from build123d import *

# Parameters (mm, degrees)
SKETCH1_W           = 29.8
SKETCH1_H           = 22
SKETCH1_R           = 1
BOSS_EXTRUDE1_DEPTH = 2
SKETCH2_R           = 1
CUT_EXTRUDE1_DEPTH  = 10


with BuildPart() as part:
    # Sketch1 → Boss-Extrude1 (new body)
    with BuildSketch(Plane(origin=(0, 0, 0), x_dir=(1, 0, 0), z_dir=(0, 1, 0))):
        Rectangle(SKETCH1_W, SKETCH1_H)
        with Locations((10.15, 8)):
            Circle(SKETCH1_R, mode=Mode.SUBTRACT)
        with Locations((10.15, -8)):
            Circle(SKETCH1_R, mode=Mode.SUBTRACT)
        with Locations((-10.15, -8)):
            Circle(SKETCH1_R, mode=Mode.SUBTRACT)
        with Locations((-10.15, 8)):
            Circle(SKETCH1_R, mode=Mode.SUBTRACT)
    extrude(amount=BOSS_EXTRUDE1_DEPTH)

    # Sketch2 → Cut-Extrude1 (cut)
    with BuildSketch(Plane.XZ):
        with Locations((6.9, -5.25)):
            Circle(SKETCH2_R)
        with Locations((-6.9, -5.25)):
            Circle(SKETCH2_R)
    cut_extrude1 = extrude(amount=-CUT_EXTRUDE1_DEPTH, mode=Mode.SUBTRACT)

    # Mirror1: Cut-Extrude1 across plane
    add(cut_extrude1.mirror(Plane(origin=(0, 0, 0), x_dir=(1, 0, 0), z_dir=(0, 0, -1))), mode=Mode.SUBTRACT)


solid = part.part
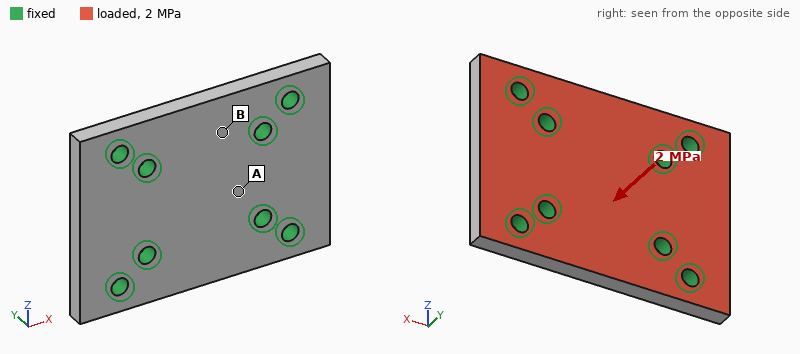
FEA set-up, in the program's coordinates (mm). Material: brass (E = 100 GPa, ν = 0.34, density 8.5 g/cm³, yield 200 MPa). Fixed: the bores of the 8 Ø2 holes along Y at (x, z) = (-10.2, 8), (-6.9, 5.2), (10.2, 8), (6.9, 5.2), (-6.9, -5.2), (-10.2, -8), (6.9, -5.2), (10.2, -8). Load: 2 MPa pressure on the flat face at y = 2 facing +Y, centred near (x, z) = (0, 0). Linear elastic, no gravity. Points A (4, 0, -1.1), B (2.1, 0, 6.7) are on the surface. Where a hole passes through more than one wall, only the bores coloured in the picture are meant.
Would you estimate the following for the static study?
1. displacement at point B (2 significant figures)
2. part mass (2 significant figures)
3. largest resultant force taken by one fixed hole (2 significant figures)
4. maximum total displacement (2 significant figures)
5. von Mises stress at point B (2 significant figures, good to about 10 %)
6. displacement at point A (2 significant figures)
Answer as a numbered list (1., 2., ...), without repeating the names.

1. 3.3 µm
2. 11 g
3. 200 N
4. 6.4 µm
5. 19 MPa
6. 2.3 µm
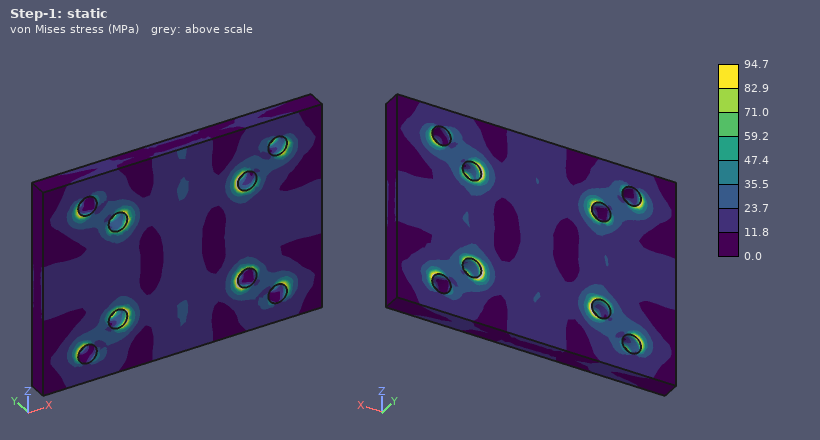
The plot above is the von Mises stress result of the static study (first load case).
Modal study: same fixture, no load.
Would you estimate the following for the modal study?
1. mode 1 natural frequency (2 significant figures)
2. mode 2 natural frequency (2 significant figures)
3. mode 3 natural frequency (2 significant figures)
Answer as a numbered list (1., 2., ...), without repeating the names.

1. 27 kHz
2. 28 kHz
3. 28 kHz
